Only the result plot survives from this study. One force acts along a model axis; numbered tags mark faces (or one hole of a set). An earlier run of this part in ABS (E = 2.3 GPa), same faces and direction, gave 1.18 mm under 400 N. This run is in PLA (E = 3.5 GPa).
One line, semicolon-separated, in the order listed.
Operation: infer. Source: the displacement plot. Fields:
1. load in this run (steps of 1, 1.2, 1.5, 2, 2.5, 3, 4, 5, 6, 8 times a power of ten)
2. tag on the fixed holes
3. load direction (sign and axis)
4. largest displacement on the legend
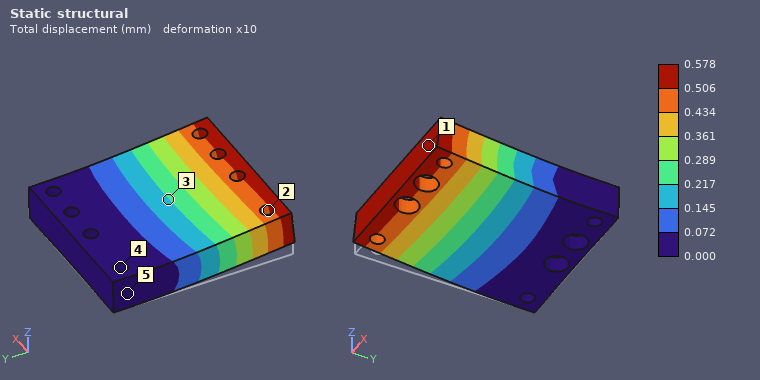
300 N; 4; +Z; 0.578 mm
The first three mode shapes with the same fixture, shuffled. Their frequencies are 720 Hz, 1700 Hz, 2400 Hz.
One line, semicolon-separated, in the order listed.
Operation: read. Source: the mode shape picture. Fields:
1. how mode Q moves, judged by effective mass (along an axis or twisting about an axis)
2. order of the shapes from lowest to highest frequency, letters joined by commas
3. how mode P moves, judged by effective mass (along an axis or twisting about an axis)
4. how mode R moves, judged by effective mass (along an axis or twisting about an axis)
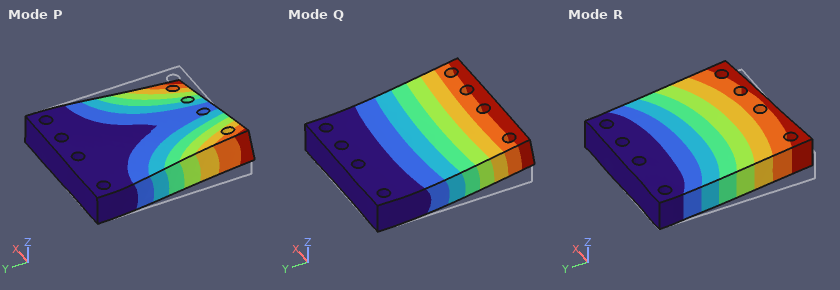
along Z; Q, P, R; twisting about Y; along X
